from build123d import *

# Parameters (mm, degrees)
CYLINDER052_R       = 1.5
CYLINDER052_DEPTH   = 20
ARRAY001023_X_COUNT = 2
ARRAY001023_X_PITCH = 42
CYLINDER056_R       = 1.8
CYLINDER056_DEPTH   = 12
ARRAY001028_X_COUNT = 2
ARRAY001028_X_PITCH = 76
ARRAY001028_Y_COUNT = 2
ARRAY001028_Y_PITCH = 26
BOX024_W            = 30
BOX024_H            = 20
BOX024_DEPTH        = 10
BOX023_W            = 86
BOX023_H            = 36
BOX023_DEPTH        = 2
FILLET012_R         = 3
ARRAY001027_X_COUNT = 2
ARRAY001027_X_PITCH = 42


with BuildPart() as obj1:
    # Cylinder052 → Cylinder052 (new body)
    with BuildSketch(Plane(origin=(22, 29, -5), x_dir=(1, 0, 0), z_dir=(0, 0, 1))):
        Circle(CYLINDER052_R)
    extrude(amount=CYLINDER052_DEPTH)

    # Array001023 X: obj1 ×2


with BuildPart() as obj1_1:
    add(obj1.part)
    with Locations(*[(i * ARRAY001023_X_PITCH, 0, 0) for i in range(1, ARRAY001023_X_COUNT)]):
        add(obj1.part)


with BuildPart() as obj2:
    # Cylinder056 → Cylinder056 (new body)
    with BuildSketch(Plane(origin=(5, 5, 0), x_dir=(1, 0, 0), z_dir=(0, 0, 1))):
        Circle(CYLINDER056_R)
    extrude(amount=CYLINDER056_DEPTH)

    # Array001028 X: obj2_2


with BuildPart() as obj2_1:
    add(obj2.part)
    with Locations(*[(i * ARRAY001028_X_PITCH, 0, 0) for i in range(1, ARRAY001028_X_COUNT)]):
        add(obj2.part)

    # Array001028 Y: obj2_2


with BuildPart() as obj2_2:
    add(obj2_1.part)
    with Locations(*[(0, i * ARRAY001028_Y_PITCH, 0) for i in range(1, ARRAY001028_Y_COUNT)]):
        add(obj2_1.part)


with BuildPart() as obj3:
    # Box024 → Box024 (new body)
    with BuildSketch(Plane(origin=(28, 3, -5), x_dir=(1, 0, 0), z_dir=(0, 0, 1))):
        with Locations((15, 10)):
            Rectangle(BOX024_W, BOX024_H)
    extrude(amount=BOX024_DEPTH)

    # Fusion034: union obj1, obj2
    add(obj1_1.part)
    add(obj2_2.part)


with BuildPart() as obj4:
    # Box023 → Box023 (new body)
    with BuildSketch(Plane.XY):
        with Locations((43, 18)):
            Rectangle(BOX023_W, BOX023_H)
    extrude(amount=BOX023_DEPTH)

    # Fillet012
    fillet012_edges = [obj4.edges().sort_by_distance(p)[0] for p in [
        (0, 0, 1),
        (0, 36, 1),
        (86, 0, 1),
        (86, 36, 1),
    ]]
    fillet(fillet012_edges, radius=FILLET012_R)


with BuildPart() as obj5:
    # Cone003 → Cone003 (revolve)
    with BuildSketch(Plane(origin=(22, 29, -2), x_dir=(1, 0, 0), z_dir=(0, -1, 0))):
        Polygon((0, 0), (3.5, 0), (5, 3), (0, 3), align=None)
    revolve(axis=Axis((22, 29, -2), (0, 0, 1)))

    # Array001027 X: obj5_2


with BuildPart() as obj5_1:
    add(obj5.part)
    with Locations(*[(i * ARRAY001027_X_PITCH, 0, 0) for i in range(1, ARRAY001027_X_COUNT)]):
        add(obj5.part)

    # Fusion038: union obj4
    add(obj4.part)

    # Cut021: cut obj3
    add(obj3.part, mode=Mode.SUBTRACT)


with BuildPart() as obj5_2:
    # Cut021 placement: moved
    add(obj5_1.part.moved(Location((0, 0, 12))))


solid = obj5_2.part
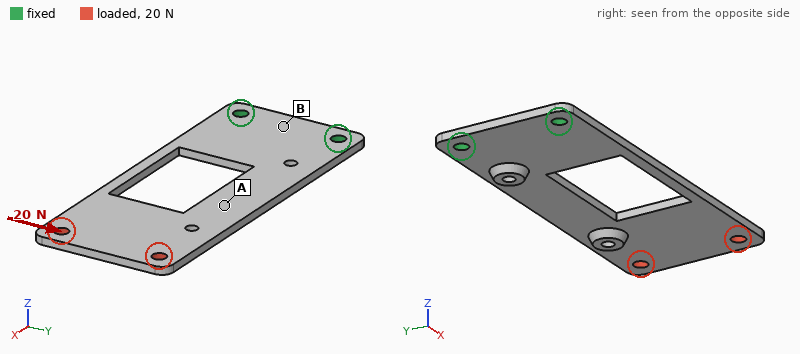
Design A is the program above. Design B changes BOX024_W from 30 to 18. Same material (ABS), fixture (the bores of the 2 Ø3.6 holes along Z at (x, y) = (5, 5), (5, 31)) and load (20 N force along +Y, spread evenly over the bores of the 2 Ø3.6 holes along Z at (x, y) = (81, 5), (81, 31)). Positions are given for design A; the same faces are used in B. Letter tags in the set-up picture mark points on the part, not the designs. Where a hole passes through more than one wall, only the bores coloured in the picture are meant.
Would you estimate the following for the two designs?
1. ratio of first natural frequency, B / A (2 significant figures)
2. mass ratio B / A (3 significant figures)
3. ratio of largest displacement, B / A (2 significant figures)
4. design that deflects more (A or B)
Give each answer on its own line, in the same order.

1.0
1.10
0.74
A
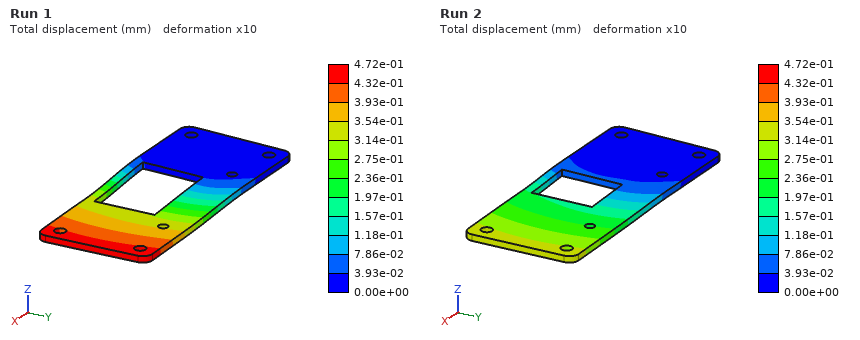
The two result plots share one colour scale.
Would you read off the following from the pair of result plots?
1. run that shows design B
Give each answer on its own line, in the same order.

Run 2
